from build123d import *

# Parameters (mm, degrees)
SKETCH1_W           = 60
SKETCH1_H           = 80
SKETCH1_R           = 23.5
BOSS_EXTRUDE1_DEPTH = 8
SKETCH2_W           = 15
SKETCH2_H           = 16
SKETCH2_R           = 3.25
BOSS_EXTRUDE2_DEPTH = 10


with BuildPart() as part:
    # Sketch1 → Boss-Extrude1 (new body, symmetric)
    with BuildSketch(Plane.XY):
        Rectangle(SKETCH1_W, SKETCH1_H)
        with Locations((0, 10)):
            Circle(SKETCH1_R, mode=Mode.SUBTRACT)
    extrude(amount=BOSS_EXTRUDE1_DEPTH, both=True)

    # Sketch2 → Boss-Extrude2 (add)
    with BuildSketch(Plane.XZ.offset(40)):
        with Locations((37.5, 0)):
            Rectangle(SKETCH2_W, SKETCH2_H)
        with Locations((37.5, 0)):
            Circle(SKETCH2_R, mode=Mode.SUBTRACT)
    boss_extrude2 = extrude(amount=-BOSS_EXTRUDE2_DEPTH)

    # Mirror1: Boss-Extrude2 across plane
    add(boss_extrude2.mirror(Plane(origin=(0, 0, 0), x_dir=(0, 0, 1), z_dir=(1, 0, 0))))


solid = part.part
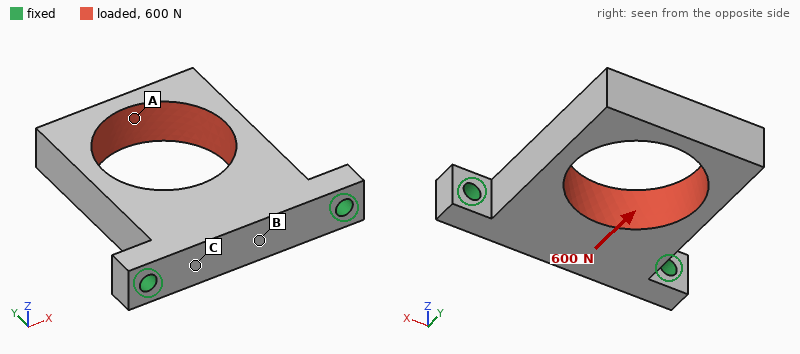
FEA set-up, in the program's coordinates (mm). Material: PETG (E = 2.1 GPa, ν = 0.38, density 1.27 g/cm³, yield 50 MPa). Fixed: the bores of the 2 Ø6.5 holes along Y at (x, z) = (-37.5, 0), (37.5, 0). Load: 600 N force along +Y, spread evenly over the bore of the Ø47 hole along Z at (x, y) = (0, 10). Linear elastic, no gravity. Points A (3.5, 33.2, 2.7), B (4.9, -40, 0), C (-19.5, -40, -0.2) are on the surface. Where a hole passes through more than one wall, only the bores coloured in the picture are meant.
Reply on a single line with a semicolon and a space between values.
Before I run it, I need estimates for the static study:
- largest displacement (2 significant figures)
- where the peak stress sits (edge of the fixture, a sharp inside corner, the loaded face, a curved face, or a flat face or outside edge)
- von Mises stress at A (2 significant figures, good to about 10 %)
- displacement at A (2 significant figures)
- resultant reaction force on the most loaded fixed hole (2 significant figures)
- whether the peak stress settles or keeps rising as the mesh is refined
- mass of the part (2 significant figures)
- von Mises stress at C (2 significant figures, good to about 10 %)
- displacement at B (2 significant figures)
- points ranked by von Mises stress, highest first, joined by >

0.16 mm; edge of the fixture; 2.3 MPa; 0.15 mm; 320 N; keeps rising; 68 g; 1.2 MPa; 0.047 mm; A > C > B
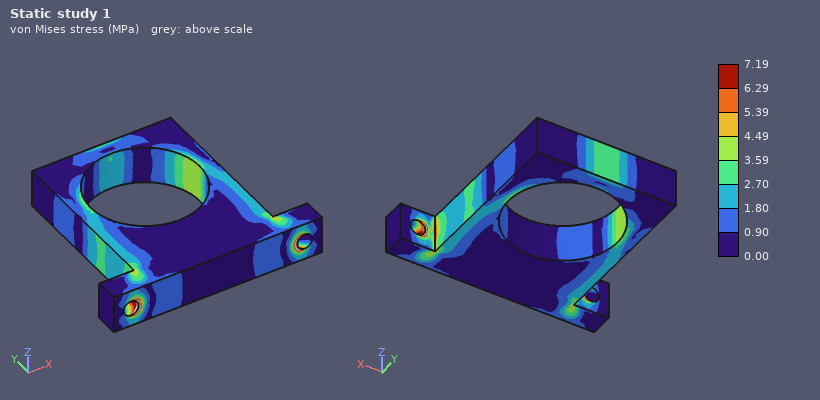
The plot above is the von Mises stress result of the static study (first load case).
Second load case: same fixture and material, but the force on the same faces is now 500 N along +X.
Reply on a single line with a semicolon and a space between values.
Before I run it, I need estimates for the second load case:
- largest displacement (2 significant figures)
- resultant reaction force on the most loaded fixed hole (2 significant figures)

0.61 mm; 430 N
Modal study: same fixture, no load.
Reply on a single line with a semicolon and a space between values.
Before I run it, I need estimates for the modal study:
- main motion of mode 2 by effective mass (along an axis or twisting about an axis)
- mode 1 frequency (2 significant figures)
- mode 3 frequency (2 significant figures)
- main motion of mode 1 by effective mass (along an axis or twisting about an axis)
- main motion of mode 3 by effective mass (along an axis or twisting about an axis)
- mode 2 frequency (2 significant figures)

along X; 320 Hz; 900 Hz; along Z; twisting about Y; 810 Hz
